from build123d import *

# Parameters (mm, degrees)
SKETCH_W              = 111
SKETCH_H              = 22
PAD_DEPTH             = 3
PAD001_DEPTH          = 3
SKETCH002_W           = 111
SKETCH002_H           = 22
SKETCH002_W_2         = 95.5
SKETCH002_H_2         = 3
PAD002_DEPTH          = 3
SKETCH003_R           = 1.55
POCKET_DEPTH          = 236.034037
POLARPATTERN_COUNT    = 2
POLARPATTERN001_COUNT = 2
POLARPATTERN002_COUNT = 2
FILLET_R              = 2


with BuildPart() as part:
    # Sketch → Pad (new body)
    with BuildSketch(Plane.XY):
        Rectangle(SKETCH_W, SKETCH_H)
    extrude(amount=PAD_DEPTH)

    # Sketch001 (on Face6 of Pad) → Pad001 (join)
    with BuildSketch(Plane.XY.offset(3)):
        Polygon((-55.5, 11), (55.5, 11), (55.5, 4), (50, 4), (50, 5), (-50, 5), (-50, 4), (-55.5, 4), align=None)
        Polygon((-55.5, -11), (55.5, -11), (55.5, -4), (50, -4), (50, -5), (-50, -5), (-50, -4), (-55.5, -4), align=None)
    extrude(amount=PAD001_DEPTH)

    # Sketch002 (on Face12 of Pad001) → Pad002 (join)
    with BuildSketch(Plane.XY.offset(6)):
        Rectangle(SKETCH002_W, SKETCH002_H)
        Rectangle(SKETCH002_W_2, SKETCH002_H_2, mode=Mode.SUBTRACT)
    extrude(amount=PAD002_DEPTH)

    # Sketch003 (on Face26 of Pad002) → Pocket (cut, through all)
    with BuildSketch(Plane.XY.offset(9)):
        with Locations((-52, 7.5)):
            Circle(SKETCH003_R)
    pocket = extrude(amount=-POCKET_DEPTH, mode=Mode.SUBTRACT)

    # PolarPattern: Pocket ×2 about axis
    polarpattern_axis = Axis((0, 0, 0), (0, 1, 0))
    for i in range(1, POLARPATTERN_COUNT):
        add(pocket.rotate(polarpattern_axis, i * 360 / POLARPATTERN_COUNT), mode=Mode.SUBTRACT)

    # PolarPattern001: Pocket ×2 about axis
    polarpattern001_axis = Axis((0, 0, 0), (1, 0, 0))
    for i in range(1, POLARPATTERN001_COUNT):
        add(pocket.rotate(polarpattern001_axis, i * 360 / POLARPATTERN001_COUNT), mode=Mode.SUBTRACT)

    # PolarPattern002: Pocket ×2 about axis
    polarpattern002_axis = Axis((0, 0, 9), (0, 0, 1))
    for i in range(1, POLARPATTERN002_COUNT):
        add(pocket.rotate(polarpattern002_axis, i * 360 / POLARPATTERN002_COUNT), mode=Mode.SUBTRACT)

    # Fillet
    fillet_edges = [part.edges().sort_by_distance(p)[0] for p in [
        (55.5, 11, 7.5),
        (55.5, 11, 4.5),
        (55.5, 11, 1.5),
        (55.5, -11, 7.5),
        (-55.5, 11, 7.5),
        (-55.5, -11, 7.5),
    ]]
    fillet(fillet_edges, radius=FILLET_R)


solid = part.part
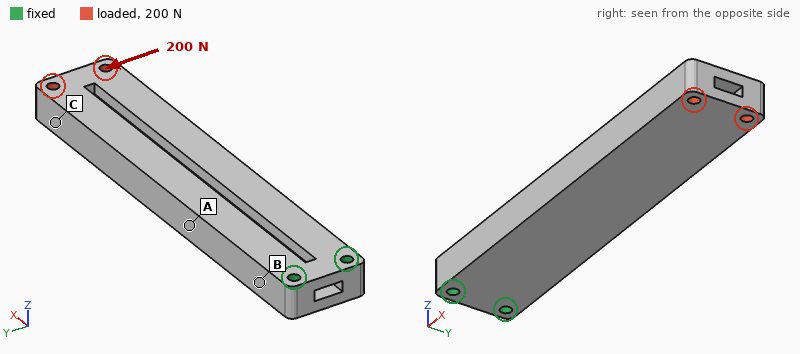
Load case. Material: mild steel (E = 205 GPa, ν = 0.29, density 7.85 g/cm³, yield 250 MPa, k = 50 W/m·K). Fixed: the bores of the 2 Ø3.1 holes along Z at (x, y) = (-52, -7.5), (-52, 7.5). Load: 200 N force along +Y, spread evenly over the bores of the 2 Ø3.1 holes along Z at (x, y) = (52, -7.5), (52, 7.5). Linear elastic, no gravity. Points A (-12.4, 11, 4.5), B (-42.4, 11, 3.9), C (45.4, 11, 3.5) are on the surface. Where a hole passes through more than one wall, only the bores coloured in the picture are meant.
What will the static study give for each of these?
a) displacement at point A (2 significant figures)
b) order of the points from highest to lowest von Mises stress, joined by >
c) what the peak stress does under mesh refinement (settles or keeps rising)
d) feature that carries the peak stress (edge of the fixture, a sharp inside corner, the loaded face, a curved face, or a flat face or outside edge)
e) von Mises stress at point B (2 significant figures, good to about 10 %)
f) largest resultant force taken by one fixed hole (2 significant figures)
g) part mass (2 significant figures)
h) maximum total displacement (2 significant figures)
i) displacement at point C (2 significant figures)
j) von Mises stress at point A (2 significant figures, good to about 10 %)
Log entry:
13 µm
B > A > C
keeps rising
edge of the fixture
29 MPa
1.3 kN
140 g
63 µm
51 µm
19 MPa
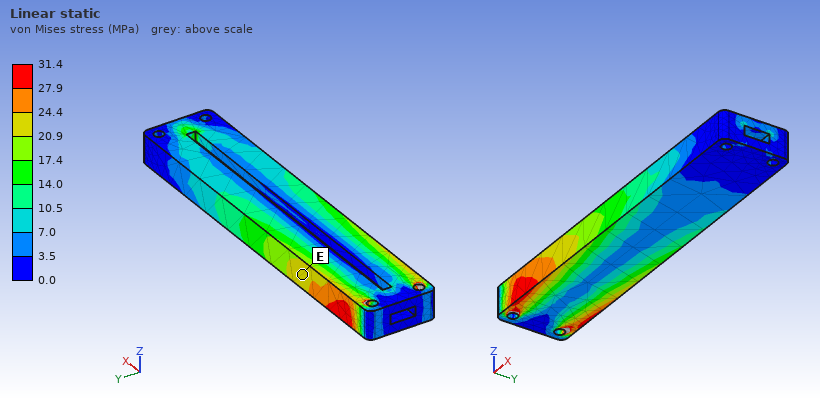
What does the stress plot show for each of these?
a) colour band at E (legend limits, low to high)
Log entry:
20.9 to 24.4 MPa
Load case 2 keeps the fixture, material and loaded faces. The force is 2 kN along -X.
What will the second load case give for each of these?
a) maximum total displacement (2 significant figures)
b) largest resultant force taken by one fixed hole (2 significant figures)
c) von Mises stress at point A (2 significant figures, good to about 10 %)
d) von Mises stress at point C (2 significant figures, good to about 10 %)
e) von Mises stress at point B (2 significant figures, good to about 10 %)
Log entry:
10 µm
1.0 kN
13 MPa
16 MPa
13 MPa
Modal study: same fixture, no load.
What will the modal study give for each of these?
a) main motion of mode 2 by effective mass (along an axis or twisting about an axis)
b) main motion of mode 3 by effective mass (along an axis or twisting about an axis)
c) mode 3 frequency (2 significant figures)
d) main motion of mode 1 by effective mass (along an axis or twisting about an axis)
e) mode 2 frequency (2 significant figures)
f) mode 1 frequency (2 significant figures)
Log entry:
along Y
twisting about X
3300 Hz
along Z
1500 Hz
680 Hz
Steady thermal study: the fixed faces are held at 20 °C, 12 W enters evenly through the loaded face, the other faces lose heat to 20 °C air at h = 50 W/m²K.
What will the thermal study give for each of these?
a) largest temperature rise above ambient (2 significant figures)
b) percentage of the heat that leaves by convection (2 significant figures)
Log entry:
60 K
84 %
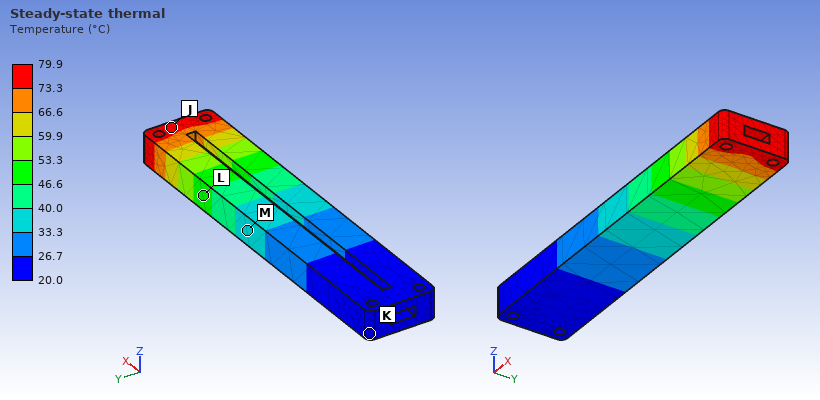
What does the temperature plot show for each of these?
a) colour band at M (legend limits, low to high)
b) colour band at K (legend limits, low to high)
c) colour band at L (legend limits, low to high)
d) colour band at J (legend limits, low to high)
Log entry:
33.3 to 40.0 °C
20.0 to 26.7 °C
46.6 to 53.3 °C
73.3 to 79.9 °C
